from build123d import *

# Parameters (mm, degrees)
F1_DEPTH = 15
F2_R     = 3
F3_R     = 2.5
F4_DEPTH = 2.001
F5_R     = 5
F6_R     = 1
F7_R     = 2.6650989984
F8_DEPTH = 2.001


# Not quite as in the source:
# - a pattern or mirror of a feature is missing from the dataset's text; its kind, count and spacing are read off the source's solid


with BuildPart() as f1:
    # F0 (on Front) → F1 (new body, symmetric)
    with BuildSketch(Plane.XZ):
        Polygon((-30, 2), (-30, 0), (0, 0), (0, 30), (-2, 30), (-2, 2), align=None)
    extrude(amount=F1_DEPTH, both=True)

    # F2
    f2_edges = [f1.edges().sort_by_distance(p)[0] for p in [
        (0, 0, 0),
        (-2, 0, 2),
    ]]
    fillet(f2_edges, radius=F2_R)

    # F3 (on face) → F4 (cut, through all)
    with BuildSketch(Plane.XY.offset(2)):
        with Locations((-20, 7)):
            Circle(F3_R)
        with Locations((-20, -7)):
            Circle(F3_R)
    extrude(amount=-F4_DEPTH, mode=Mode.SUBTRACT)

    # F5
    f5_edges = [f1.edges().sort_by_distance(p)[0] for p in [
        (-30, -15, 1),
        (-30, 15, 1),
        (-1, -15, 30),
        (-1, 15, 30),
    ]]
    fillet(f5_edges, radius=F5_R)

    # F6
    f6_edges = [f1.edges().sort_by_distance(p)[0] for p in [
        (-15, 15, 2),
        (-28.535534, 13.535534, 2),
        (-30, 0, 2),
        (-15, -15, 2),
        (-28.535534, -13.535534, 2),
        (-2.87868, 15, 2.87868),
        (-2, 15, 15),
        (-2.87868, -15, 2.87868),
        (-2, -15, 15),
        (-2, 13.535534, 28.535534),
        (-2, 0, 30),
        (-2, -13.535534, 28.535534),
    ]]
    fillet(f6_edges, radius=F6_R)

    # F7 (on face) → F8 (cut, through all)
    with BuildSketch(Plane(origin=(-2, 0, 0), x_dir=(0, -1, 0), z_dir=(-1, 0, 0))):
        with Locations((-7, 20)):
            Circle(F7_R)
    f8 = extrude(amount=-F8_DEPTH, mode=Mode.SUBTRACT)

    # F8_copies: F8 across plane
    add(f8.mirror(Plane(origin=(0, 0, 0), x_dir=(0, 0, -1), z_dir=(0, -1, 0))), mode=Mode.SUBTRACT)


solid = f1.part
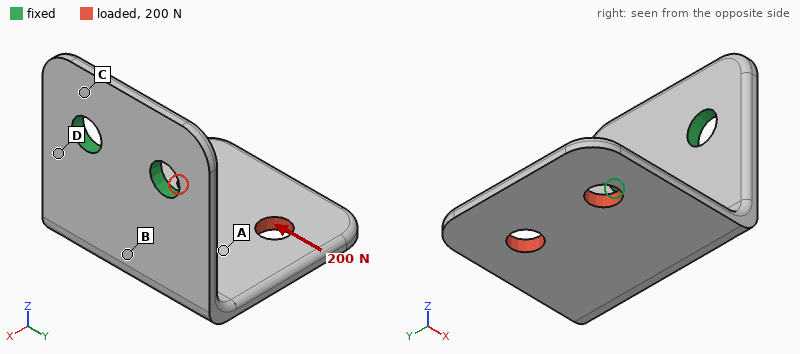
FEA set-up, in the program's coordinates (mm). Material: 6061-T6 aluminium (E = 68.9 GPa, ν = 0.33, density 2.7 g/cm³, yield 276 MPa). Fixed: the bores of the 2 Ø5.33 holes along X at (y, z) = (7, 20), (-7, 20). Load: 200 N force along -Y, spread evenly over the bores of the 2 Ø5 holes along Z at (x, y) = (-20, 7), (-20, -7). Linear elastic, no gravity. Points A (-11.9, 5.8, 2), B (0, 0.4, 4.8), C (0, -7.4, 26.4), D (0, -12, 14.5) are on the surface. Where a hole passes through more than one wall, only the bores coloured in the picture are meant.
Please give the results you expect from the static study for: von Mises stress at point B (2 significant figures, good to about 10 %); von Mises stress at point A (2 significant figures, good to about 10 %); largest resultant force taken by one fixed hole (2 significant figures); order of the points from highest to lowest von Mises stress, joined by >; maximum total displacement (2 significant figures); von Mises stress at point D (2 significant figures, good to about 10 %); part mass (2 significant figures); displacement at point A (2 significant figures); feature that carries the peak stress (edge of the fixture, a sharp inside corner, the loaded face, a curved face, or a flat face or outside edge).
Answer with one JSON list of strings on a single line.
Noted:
["78 MPa", "29 MPa", "300 N", "D > B > A > C", "0.44 mm", "97 MPa", "8.7 g", "0.18 mm", "a flat face or outside edge"]
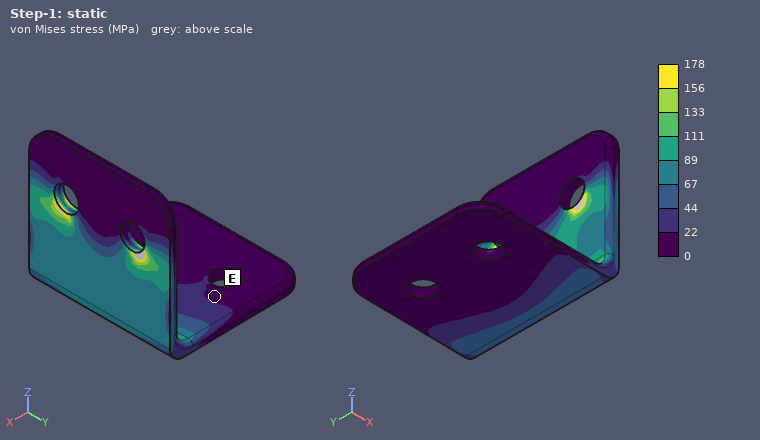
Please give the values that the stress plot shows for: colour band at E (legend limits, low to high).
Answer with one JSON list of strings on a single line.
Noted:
["0 to 22 MPa"]
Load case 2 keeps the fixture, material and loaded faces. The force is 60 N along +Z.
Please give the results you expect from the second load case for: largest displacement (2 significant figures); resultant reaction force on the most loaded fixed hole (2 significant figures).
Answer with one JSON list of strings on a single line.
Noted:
["0.50 mm", "32 N"]
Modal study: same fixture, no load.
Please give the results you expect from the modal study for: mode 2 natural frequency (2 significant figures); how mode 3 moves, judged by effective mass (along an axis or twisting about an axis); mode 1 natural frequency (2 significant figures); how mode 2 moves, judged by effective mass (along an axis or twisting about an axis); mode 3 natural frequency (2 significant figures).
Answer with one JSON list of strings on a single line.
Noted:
["2100 Hz", "along X", "1100 Hz", "along Y", "3500 Hz"]
